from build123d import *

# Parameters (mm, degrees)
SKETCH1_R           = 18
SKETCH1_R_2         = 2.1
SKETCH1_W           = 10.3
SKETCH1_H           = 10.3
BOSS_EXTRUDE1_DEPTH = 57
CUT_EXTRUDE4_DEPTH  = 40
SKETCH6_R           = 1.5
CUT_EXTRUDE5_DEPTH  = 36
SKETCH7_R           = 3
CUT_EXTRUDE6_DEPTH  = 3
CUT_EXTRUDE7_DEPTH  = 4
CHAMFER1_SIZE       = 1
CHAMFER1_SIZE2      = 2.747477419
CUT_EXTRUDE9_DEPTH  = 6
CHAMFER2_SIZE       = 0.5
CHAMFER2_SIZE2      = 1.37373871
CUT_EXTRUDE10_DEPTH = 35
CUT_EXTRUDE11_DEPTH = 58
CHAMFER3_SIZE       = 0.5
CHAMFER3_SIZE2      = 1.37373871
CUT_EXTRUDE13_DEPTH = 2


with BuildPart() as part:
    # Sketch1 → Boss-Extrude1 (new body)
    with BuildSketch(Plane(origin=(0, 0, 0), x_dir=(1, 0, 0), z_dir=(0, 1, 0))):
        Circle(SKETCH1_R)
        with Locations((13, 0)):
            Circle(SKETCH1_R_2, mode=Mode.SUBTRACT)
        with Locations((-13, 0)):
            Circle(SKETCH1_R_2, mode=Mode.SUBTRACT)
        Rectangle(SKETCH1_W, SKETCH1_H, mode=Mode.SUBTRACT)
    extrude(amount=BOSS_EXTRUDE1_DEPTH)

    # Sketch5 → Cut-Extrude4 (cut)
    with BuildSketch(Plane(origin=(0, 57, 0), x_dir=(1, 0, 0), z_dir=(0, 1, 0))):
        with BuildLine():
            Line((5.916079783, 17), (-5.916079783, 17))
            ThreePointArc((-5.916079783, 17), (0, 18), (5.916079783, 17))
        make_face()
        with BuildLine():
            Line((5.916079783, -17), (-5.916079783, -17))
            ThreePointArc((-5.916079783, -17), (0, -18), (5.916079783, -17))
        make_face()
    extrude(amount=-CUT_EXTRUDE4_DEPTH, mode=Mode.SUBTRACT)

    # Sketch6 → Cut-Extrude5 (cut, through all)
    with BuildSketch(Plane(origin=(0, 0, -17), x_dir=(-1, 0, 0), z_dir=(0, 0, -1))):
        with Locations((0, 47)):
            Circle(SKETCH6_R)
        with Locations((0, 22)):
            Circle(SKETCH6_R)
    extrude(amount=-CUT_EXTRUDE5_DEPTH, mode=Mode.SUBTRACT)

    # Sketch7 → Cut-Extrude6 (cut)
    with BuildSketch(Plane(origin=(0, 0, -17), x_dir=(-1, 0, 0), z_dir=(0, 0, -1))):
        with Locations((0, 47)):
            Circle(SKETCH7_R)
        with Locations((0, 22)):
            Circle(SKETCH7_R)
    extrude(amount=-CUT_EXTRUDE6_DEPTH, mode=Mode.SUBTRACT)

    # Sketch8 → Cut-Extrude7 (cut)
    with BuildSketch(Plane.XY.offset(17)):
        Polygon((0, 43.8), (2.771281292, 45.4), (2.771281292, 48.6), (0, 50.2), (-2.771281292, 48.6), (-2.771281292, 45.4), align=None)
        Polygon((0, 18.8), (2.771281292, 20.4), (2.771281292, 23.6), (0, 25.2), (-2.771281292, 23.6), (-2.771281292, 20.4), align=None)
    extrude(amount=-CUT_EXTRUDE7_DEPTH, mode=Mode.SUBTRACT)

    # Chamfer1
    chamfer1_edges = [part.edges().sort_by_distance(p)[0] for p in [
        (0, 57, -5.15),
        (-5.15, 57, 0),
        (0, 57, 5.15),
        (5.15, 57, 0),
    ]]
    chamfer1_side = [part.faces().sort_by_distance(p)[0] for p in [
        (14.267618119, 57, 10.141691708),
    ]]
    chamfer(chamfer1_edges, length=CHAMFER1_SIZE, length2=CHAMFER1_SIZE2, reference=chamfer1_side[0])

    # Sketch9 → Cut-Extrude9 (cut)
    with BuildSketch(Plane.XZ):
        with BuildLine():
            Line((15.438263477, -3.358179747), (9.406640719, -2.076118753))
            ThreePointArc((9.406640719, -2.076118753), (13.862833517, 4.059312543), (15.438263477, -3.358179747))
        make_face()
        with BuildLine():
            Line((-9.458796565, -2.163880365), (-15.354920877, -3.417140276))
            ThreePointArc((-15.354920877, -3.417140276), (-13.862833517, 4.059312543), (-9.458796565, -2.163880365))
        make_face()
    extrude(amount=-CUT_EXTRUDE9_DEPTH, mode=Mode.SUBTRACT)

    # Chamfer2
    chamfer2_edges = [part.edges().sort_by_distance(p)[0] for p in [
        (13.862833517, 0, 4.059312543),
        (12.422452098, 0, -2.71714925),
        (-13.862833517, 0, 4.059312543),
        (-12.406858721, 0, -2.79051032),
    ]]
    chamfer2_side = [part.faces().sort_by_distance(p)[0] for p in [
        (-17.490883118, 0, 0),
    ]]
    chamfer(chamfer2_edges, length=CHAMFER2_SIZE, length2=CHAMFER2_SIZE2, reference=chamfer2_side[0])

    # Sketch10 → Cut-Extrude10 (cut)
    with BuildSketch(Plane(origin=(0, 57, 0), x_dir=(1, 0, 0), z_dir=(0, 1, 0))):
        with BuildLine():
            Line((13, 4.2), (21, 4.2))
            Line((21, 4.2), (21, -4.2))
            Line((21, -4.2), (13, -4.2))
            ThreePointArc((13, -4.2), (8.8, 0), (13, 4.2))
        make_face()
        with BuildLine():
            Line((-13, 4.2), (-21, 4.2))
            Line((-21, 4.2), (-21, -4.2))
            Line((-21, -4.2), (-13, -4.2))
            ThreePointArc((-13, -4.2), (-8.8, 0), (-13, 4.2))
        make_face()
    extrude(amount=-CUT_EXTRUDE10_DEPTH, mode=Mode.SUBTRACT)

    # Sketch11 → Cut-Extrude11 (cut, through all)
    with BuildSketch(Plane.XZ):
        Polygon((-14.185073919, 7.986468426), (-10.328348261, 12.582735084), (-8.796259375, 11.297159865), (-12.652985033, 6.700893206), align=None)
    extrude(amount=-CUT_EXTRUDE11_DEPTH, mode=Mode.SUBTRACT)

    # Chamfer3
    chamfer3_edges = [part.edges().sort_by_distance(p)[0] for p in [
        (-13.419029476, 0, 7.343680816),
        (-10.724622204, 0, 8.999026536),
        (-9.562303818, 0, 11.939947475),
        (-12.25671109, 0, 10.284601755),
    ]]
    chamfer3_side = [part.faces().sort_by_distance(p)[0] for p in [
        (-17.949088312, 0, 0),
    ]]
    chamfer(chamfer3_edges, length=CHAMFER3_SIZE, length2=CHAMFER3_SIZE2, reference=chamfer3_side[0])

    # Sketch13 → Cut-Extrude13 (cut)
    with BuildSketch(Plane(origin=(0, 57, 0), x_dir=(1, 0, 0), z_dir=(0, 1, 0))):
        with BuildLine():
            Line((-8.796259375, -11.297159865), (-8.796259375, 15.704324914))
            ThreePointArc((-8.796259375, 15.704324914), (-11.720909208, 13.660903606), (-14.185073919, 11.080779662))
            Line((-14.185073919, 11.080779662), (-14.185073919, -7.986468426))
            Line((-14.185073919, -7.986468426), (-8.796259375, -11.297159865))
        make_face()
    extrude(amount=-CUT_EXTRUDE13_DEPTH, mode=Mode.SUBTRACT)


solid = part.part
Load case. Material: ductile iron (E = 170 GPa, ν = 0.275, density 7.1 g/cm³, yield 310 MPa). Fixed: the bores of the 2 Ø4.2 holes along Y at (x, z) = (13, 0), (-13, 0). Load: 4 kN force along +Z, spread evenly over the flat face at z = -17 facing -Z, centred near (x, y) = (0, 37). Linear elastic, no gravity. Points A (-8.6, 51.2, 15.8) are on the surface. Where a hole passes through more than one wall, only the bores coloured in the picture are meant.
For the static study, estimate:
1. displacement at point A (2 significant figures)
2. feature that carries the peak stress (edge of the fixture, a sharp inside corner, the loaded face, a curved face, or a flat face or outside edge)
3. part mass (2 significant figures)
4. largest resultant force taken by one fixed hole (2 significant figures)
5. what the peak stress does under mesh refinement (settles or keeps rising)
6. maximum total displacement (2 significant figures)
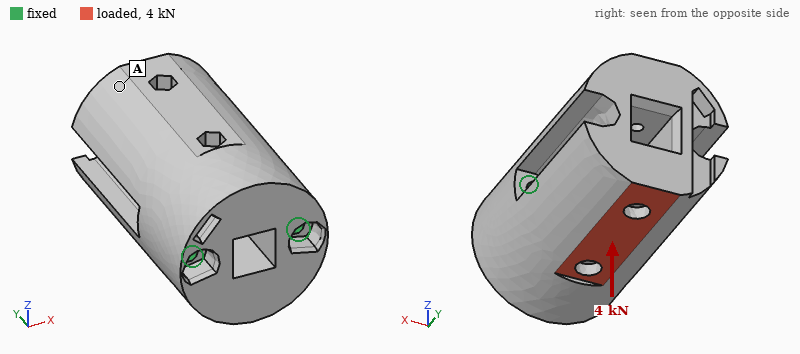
18 µm
edge of the fixture
310 g
2.0 kN
keeps rising
22 µm
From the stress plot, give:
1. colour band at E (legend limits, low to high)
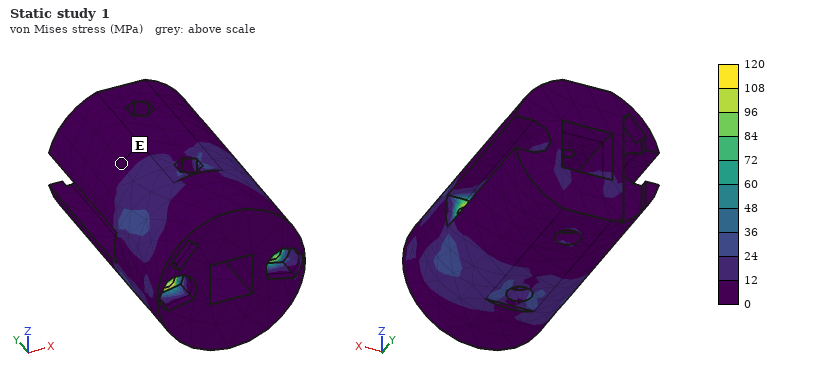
0 to 12 MPa
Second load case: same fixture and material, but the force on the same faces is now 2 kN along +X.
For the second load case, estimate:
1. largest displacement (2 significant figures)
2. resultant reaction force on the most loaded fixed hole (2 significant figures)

6.8 µm
2.2 kN
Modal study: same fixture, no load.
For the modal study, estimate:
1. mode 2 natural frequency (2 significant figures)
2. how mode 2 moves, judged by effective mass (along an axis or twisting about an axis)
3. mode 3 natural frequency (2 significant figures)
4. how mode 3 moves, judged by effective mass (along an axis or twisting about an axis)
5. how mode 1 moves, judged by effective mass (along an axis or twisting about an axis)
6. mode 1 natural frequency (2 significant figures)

9100 Hz
along X
15 kHz
twisting about Y
along Z
5800 Hz
